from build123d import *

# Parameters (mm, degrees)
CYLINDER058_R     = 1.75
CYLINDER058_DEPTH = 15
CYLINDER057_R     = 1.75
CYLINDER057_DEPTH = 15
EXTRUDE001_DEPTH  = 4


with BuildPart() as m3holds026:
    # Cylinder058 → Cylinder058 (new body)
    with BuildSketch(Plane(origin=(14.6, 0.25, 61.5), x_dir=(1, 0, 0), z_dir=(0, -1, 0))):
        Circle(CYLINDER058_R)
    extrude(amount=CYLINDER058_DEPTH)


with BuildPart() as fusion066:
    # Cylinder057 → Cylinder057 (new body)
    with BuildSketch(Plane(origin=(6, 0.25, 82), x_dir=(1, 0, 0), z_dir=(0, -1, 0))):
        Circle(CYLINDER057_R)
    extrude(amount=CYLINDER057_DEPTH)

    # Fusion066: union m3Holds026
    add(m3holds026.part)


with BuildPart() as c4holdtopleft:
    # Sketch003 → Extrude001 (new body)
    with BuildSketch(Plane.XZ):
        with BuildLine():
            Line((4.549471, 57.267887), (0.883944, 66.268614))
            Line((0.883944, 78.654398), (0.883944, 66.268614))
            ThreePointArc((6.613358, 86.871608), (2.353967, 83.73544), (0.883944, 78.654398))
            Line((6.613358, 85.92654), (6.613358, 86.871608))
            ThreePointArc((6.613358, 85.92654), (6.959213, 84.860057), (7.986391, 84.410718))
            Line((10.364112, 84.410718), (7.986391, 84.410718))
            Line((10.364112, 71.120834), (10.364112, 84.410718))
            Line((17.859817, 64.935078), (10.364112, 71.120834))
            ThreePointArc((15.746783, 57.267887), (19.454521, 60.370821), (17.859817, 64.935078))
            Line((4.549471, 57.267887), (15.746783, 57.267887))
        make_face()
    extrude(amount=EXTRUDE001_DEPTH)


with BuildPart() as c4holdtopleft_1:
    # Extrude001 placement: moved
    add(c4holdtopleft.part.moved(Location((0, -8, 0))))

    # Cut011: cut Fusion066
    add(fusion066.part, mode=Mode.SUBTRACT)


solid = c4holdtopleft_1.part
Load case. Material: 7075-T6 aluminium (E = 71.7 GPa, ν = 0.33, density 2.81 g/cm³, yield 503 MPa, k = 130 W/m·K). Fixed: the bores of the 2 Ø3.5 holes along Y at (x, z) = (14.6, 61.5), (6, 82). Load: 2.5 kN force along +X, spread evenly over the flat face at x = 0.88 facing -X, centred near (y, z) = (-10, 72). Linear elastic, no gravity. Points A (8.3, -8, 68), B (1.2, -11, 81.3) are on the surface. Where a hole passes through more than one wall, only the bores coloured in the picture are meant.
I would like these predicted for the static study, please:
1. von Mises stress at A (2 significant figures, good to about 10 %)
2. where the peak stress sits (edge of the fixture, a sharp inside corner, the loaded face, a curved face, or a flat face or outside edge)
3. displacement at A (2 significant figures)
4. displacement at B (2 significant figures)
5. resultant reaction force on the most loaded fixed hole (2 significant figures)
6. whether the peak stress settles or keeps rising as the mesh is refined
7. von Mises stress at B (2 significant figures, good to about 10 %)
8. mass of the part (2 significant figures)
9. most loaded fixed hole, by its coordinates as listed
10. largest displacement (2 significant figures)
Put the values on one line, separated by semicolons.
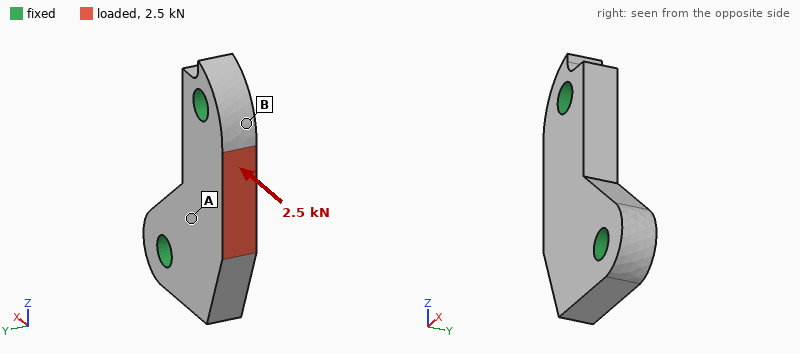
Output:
55 MPa; edge of the fixture; 8.3 µm; 3.1 µm; 1.5 kN; keeps rising; 30 MPa; 3.5 g; (14.6, 61.5); 14 µm
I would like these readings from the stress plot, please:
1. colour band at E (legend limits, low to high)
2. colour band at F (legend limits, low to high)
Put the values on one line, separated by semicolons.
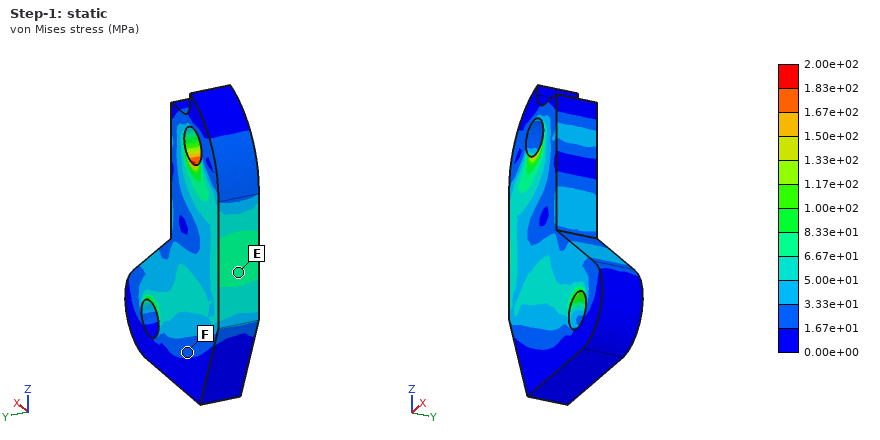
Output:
6.67e+01 to 8.33e+01 MPa; 1.67e+01 to 3.33e+01 MPa
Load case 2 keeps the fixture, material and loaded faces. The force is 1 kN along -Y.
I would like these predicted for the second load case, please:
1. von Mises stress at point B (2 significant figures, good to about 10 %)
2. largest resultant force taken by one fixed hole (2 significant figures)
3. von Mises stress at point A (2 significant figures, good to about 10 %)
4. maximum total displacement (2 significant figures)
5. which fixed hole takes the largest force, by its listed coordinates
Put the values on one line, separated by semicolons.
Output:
46 MPa; 730 N; 71 MPa; 66 µm; (6, 82)
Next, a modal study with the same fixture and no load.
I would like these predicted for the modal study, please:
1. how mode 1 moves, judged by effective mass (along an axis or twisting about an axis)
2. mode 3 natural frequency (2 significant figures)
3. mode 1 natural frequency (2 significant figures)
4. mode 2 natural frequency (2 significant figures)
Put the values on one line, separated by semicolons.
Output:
along Y; 55 kHz; 24 kHz; 46 kHz
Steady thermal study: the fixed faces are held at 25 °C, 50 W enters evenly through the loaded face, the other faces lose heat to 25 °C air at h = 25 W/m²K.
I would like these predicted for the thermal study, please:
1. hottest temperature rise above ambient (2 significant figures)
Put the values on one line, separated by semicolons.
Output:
65 K
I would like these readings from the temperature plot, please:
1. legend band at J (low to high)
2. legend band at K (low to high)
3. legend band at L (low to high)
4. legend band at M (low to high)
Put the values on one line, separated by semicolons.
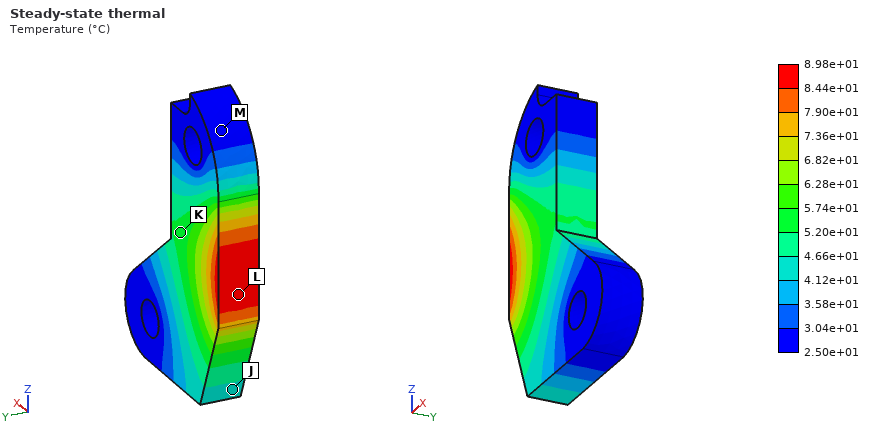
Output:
4.12e+01 to 4.66e+01 °C; 5.20e+01 to 5.74e+01 °C; 8.44e+01 to 8.98e+01 °C; 2.50e+01 to 3.04e+01 °C
